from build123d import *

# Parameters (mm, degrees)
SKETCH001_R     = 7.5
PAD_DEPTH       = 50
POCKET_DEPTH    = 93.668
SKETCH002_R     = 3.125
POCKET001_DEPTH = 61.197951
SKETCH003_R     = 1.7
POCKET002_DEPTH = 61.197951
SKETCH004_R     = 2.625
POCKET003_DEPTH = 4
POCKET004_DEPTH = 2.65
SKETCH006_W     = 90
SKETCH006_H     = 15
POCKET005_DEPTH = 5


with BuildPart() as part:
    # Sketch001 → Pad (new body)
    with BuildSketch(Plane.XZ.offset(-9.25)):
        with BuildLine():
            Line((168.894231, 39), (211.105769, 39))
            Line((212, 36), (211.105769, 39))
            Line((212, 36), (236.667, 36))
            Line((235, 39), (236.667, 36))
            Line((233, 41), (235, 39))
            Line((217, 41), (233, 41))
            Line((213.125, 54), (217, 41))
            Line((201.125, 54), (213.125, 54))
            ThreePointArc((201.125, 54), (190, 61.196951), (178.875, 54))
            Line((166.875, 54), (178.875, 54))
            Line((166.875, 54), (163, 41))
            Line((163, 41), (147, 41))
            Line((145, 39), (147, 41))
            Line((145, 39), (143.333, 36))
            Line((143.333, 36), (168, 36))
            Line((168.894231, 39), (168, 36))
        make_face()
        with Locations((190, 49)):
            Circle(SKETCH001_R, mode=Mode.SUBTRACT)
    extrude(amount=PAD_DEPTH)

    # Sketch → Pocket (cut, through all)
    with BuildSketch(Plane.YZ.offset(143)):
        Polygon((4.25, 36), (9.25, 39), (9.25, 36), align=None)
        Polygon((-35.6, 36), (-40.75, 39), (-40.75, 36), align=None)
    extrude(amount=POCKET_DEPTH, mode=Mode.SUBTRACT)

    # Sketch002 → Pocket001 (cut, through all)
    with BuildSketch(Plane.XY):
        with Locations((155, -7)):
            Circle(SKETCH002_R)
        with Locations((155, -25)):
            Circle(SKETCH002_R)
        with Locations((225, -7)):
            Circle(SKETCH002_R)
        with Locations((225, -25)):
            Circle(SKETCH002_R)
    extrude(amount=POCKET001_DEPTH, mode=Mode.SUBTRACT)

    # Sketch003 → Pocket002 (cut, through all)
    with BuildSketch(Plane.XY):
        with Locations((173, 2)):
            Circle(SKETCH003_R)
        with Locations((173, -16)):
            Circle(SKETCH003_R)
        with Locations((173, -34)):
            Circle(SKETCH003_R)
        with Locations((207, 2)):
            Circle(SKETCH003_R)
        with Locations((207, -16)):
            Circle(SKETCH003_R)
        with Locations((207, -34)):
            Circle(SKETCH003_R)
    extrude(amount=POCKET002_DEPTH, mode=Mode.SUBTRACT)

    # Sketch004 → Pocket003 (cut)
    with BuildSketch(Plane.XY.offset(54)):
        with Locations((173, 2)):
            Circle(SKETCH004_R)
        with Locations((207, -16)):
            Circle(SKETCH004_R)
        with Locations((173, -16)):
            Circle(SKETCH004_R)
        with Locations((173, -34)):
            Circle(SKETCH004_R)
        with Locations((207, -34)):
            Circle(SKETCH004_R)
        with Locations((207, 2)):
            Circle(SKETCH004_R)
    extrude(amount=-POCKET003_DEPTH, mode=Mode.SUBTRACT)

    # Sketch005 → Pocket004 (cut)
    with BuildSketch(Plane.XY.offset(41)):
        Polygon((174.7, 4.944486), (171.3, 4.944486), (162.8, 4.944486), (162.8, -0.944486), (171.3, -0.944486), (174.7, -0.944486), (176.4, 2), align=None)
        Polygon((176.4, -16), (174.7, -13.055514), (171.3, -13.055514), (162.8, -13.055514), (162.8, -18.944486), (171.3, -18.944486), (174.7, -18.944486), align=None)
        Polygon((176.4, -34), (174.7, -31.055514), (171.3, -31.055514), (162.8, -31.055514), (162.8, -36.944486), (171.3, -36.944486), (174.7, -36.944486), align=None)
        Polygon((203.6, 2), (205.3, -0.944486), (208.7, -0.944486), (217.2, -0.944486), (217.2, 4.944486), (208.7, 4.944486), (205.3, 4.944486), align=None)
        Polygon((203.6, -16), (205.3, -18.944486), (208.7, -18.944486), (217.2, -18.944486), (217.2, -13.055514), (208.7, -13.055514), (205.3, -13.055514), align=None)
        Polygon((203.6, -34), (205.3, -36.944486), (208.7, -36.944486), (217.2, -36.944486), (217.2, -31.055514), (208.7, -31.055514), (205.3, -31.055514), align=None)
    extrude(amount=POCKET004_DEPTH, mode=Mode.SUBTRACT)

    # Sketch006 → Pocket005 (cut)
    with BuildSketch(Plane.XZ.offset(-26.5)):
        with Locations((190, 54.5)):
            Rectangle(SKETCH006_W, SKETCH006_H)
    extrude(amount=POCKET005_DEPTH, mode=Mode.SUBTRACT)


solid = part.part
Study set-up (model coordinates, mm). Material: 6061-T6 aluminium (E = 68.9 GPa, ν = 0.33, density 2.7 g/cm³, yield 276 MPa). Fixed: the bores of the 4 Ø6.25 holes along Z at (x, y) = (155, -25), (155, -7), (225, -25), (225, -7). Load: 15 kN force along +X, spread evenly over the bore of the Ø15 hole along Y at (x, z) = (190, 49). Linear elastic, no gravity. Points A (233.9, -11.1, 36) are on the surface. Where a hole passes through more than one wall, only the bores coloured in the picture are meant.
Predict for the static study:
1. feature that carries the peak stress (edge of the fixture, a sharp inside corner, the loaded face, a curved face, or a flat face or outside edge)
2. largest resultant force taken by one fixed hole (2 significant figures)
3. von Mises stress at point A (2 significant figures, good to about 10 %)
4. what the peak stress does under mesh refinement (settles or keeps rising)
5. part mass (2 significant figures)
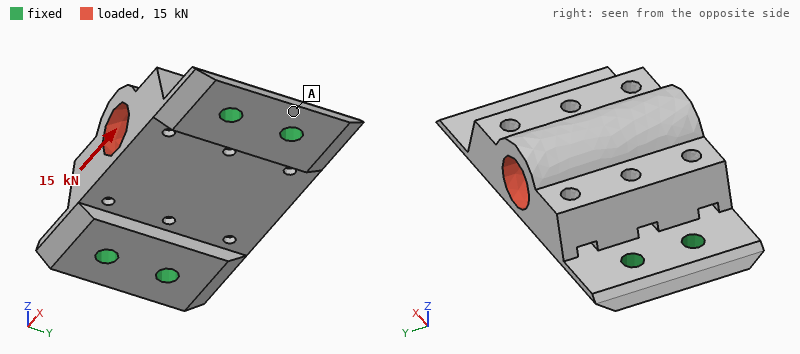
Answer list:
edge of the fixture
4.0 kN
14 MPa
keeps rising
110 g
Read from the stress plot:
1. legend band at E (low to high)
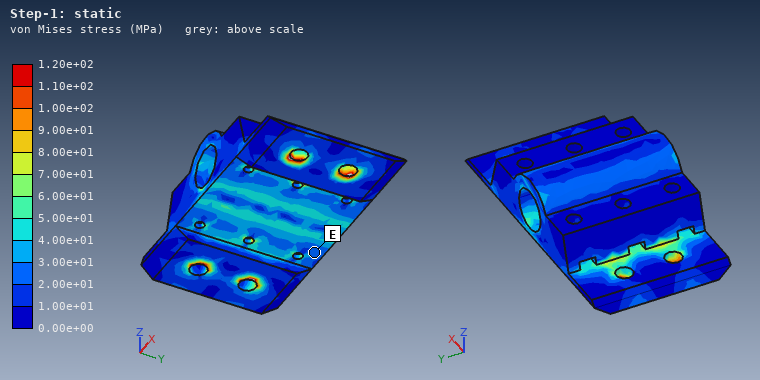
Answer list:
2.00e+01 to 3.00e+01 MPa
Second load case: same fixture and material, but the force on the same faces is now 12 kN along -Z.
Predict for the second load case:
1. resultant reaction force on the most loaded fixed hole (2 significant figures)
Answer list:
4.4 kN
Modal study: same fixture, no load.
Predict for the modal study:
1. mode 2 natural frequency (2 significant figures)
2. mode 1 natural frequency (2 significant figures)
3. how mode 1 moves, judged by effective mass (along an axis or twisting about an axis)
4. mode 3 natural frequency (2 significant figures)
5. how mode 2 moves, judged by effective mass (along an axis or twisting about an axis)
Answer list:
8100 Hz
5600 Hz
along Y
13 kHz
along Z
